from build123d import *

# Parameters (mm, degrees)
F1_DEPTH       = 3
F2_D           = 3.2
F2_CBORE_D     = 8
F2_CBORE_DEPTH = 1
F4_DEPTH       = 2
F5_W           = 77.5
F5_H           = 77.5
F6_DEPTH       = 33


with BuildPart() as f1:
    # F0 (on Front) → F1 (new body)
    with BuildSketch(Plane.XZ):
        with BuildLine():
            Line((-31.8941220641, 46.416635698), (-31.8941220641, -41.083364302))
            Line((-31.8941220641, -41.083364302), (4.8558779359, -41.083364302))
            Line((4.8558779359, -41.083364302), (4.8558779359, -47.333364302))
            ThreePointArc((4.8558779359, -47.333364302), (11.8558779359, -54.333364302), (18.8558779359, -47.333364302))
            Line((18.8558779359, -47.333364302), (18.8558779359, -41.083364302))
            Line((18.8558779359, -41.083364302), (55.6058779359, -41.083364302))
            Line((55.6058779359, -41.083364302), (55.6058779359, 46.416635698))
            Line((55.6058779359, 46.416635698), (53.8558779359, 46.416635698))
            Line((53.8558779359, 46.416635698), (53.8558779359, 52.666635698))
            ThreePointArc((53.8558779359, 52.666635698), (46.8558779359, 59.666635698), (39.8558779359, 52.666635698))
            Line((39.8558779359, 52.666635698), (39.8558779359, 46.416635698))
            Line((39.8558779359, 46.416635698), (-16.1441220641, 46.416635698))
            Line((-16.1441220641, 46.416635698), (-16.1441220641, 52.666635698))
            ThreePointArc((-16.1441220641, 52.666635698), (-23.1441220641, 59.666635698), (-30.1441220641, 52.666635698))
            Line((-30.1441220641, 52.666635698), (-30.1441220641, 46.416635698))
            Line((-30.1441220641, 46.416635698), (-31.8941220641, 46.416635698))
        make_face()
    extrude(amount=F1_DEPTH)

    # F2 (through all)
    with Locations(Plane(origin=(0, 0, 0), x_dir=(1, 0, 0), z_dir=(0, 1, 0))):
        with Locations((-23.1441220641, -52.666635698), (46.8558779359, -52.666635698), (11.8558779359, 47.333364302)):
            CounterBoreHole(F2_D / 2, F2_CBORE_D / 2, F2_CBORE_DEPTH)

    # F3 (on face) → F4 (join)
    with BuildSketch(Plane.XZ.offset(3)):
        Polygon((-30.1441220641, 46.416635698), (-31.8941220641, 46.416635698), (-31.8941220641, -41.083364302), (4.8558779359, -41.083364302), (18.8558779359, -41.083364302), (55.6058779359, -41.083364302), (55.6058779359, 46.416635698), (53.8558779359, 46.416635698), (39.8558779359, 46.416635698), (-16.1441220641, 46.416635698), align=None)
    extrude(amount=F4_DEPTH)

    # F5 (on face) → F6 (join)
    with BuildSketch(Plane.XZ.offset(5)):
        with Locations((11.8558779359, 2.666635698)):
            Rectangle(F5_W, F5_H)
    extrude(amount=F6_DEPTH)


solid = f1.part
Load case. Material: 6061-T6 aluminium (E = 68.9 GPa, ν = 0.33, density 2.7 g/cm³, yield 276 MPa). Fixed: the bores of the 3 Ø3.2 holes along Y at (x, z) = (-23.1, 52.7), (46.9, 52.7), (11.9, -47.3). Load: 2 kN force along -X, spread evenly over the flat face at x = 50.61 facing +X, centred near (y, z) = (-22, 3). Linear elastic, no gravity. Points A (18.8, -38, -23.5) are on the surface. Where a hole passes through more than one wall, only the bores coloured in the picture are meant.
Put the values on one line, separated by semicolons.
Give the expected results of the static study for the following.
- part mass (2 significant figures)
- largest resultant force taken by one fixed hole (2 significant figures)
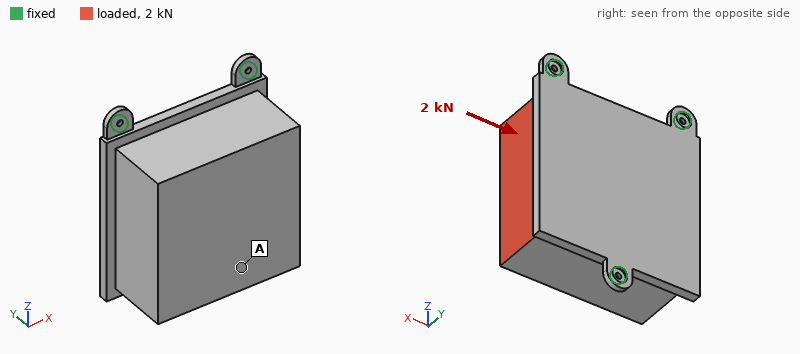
640 g; 940 N
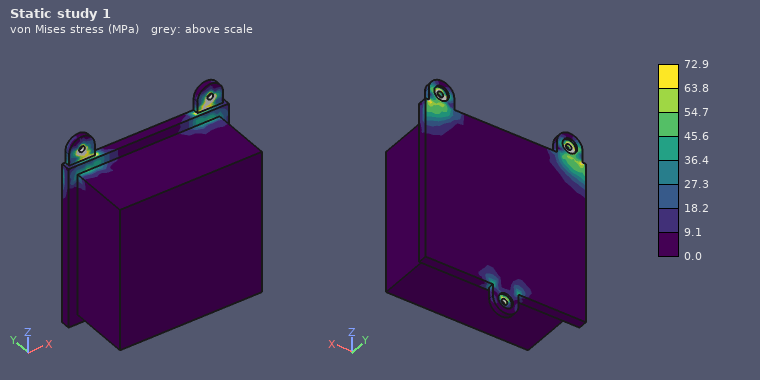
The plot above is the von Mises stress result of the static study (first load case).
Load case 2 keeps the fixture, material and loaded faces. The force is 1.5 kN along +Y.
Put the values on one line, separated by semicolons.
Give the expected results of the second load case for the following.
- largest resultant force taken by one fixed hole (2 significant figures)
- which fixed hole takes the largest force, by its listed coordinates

1.3 kN; (46.9, 52.7)
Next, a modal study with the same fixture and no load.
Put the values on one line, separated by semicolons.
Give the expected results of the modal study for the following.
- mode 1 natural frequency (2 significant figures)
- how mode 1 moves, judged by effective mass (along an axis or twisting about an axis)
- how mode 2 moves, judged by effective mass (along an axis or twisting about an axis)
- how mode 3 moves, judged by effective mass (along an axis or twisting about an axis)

1200 Hz; along X; along Y; along Z
